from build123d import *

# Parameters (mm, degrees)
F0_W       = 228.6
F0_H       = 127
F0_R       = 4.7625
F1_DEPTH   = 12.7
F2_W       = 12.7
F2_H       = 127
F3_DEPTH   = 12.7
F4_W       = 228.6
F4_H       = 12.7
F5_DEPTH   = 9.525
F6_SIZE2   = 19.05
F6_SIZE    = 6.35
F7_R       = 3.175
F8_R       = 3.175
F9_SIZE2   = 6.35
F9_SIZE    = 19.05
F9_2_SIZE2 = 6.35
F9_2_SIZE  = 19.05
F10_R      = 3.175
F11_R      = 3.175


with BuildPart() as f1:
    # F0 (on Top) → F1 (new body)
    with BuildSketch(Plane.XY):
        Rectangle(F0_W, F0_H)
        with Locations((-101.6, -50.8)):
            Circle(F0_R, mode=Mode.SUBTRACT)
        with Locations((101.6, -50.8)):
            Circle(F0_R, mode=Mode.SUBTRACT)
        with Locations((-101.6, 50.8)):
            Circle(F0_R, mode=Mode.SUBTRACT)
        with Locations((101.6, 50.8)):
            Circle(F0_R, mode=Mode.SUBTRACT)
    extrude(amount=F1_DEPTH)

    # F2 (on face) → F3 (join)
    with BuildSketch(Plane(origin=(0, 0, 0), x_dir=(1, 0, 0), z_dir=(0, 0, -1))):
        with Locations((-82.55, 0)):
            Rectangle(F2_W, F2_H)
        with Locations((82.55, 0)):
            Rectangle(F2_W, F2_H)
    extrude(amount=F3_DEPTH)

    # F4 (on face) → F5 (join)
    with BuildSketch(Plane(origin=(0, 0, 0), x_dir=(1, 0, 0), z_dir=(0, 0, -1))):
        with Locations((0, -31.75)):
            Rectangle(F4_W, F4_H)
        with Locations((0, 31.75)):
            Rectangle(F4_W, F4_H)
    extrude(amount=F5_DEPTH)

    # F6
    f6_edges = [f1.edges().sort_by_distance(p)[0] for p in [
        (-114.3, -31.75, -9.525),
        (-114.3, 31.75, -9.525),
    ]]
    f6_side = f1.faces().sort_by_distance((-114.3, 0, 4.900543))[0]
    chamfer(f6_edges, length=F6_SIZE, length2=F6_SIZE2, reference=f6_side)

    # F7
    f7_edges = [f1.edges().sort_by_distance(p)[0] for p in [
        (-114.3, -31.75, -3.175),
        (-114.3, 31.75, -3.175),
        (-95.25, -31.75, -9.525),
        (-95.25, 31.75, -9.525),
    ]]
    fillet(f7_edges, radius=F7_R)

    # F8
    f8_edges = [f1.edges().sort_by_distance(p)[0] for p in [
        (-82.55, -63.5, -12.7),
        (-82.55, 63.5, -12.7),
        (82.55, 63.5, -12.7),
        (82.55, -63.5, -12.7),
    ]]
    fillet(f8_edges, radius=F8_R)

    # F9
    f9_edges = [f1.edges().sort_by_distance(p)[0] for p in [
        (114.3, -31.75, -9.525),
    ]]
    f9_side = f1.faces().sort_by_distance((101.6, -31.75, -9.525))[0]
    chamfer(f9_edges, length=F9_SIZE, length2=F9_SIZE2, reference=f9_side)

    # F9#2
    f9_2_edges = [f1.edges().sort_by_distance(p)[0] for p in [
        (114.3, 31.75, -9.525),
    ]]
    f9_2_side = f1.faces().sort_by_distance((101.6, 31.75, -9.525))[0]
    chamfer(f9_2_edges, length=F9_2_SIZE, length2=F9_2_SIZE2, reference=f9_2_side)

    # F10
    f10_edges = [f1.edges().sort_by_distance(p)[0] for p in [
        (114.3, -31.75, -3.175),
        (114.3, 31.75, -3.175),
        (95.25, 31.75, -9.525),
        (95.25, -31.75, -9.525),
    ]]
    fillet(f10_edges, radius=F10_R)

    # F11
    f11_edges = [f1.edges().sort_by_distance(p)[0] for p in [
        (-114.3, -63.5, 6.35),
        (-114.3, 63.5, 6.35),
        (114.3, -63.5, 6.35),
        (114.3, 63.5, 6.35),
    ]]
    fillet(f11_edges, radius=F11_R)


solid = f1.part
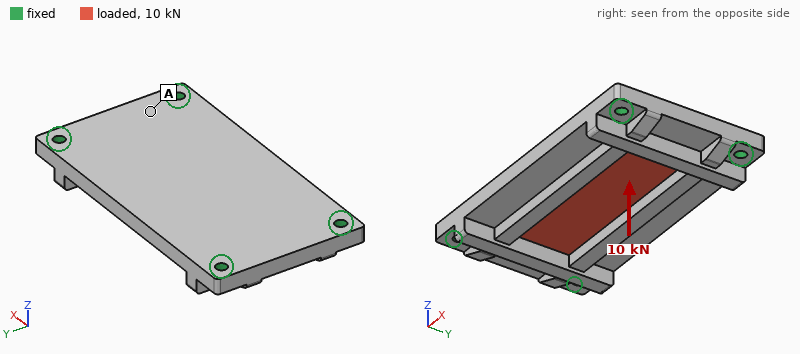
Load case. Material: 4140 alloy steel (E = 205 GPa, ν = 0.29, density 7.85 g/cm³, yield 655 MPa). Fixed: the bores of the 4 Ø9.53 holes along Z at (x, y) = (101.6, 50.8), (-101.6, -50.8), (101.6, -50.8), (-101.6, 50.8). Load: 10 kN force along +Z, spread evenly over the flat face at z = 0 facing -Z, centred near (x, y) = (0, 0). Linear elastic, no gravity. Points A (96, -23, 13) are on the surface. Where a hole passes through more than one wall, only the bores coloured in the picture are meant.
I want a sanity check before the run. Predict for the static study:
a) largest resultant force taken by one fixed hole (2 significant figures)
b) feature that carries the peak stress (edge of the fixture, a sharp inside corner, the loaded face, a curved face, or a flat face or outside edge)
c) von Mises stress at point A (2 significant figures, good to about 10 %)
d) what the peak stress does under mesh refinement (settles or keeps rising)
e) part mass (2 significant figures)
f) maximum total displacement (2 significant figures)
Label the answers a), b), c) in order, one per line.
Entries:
a) 2.9 kN
b) edge of the fixture
c) 15 MPa
d) keeps rising
e) 3.5 kg
f) 59 µm
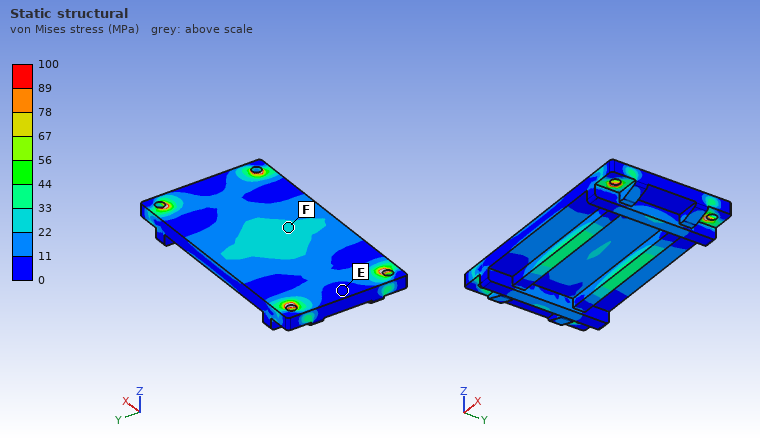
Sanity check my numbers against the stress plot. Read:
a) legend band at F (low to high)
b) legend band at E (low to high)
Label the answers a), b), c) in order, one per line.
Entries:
a) 22 to 33 MPa
b) 0 to 11 MPa
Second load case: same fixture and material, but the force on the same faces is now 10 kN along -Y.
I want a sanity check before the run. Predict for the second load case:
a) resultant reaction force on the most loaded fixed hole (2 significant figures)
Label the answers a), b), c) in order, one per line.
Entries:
a) 3.2 kN
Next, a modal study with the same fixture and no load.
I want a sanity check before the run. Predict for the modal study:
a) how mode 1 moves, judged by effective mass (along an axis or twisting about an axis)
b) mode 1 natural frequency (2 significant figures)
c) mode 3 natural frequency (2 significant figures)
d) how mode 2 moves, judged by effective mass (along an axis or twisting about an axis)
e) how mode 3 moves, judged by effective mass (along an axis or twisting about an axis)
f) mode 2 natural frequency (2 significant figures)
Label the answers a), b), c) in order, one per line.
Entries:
a) along Z
b) 1600 Hz
c) 4200 Hz
d) twisting about X
e) twisting about Y
f) 2600 Hz
